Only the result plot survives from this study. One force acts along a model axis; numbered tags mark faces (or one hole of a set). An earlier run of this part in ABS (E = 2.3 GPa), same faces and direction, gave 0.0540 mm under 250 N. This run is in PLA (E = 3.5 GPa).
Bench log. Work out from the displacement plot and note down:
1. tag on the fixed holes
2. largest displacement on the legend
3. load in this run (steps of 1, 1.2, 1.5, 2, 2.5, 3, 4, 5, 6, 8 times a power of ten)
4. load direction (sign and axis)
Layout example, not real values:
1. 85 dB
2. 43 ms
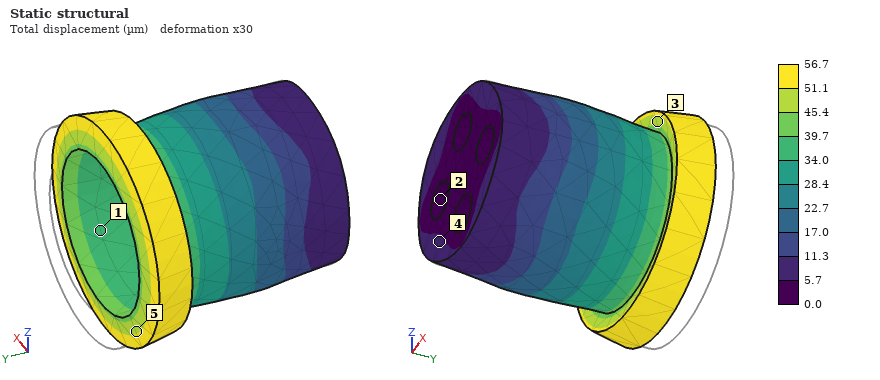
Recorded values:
1. 2
2. 56.7 µm
3. 400 N
4. -Y
